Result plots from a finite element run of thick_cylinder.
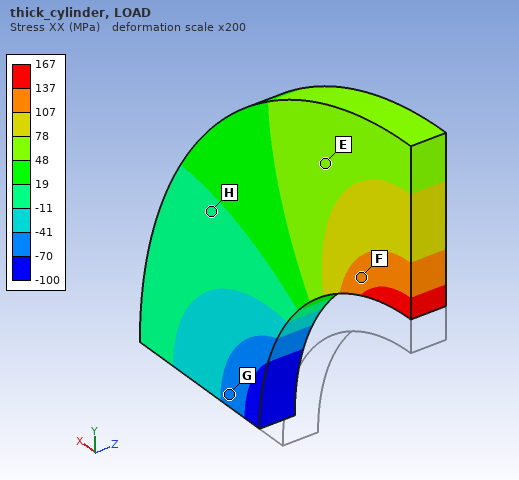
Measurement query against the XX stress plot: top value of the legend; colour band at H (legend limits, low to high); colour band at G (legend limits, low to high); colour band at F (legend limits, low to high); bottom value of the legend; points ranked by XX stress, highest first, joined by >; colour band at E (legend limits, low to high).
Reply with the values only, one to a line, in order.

167 MPa
-11 to 19 MPa
-70 to -41 MPa
107 to 137 MPa
-100 MPa
F > E > H > G
48 to 78 MPa
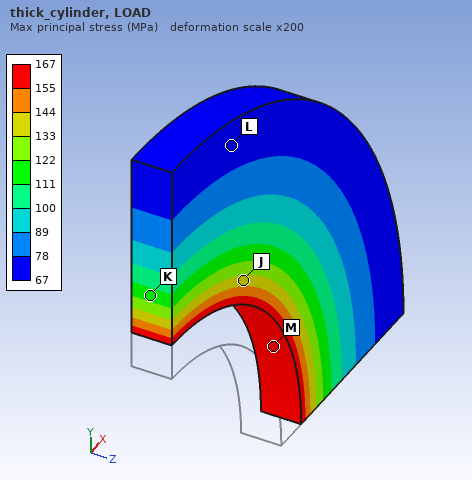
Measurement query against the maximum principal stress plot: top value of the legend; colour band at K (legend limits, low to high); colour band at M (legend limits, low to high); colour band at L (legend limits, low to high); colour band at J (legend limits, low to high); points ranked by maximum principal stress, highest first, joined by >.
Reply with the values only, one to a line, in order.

167 MPa
111 to 122 MPa
155 to 167 MPa
67 to 78 MPa
133 to 144 MPa
M > J > K > L
